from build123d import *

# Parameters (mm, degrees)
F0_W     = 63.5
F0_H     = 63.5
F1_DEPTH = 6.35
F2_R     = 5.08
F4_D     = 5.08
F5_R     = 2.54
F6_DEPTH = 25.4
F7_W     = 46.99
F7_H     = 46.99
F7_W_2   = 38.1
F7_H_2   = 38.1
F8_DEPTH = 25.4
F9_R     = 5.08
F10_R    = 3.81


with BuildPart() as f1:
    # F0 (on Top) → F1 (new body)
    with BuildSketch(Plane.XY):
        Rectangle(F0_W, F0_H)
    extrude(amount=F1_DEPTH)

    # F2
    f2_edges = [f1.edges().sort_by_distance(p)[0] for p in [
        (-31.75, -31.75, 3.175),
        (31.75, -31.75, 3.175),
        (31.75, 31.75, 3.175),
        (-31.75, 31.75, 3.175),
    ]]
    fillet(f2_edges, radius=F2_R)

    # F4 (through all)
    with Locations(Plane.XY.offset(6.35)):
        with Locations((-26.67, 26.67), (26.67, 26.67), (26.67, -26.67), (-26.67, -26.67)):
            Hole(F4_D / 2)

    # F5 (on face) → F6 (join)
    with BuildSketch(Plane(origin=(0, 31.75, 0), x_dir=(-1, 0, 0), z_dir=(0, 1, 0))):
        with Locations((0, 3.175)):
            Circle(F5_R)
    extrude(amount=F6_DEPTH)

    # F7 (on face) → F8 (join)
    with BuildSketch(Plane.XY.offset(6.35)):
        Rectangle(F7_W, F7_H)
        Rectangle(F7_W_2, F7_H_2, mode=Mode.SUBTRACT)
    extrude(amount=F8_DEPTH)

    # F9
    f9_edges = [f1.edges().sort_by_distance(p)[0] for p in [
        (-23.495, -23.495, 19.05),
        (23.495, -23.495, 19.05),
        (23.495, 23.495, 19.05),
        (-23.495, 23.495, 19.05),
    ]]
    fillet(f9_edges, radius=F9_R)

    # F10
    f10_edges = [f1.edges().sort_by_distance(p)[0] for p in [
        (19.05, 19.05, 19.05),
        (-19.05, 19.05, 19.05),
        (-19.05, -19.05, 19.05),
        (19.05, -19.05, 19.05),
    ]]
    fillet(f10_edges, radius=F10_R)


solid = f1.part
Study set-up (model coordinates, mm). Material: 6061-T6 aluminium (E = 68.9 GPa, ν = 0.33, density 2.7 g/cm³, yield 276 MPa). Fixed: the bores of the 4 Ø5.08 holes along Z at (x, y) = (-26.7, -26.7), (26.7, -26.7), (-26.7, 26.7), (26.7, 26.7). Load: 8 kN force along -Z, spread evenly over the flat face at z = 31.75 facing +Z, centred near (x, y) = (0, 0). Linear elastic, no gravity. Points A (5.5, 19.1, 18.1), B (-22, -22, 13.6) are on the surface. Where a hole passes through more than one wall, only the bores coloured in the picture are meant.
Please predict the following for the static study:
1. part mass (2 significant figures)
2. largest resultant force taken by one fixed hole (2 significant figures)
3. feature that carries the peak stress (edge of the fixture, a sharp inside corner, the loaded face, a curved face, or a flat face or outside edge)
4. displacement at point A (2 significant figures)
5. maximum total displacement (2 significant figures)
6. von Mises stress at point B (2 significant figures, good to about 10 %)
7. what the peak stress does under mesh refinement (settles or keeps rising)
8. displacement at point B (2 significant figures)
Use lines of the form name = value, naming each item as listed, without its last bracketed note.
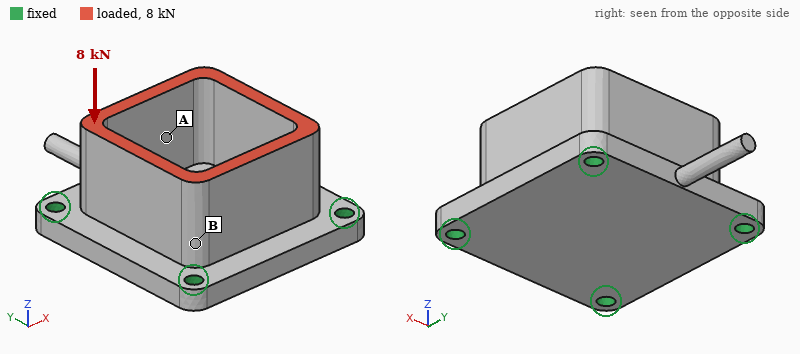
part mass = 120 g
largest resultant force taken by one fixed hole = 2.1 kN
feature that carries the peak stress = edge of the fixture
displacement at point A = 20 µm
maximum total displacement = 25 µm
von Mises stress at point B = 28 MPa
what the peak stress does under mesh refinement = keeps rising
displacement at point B = 18 µm
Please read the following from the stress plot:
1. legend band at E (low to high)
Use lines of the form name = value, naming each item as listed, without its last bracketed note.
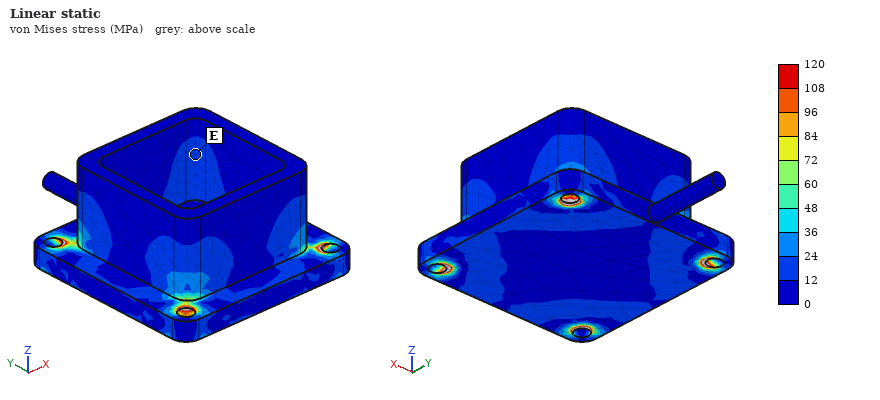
legend band at E = 12 to 24 MPa
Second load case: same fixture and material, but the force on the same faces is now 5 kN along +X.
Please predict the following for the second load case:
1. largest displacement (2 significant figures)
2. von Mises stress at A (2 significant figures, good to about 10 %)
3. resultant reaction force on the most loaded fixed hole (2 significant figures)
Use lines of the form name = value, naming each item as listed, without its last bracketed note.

largest displacement = 97 µm
von Mises stress at A = 20 MPa
resultant reaction force on the most loaded fixed hole = 2.0 kN
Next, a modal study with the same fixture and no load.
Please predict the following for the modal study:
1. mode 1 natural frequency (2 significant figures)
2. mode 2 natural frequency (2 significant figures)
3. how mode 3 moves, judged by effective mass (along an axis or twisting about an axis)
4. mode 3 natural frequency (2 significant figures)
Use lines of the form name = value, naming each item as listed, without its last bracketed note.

mode 1 natural frequency = 4500 Hz
mode 2 natural frequency = 5000 Hz
how mode 3 moves, judged by effective mass = along Z
mode 3 natural frequency = 9300 Hz
